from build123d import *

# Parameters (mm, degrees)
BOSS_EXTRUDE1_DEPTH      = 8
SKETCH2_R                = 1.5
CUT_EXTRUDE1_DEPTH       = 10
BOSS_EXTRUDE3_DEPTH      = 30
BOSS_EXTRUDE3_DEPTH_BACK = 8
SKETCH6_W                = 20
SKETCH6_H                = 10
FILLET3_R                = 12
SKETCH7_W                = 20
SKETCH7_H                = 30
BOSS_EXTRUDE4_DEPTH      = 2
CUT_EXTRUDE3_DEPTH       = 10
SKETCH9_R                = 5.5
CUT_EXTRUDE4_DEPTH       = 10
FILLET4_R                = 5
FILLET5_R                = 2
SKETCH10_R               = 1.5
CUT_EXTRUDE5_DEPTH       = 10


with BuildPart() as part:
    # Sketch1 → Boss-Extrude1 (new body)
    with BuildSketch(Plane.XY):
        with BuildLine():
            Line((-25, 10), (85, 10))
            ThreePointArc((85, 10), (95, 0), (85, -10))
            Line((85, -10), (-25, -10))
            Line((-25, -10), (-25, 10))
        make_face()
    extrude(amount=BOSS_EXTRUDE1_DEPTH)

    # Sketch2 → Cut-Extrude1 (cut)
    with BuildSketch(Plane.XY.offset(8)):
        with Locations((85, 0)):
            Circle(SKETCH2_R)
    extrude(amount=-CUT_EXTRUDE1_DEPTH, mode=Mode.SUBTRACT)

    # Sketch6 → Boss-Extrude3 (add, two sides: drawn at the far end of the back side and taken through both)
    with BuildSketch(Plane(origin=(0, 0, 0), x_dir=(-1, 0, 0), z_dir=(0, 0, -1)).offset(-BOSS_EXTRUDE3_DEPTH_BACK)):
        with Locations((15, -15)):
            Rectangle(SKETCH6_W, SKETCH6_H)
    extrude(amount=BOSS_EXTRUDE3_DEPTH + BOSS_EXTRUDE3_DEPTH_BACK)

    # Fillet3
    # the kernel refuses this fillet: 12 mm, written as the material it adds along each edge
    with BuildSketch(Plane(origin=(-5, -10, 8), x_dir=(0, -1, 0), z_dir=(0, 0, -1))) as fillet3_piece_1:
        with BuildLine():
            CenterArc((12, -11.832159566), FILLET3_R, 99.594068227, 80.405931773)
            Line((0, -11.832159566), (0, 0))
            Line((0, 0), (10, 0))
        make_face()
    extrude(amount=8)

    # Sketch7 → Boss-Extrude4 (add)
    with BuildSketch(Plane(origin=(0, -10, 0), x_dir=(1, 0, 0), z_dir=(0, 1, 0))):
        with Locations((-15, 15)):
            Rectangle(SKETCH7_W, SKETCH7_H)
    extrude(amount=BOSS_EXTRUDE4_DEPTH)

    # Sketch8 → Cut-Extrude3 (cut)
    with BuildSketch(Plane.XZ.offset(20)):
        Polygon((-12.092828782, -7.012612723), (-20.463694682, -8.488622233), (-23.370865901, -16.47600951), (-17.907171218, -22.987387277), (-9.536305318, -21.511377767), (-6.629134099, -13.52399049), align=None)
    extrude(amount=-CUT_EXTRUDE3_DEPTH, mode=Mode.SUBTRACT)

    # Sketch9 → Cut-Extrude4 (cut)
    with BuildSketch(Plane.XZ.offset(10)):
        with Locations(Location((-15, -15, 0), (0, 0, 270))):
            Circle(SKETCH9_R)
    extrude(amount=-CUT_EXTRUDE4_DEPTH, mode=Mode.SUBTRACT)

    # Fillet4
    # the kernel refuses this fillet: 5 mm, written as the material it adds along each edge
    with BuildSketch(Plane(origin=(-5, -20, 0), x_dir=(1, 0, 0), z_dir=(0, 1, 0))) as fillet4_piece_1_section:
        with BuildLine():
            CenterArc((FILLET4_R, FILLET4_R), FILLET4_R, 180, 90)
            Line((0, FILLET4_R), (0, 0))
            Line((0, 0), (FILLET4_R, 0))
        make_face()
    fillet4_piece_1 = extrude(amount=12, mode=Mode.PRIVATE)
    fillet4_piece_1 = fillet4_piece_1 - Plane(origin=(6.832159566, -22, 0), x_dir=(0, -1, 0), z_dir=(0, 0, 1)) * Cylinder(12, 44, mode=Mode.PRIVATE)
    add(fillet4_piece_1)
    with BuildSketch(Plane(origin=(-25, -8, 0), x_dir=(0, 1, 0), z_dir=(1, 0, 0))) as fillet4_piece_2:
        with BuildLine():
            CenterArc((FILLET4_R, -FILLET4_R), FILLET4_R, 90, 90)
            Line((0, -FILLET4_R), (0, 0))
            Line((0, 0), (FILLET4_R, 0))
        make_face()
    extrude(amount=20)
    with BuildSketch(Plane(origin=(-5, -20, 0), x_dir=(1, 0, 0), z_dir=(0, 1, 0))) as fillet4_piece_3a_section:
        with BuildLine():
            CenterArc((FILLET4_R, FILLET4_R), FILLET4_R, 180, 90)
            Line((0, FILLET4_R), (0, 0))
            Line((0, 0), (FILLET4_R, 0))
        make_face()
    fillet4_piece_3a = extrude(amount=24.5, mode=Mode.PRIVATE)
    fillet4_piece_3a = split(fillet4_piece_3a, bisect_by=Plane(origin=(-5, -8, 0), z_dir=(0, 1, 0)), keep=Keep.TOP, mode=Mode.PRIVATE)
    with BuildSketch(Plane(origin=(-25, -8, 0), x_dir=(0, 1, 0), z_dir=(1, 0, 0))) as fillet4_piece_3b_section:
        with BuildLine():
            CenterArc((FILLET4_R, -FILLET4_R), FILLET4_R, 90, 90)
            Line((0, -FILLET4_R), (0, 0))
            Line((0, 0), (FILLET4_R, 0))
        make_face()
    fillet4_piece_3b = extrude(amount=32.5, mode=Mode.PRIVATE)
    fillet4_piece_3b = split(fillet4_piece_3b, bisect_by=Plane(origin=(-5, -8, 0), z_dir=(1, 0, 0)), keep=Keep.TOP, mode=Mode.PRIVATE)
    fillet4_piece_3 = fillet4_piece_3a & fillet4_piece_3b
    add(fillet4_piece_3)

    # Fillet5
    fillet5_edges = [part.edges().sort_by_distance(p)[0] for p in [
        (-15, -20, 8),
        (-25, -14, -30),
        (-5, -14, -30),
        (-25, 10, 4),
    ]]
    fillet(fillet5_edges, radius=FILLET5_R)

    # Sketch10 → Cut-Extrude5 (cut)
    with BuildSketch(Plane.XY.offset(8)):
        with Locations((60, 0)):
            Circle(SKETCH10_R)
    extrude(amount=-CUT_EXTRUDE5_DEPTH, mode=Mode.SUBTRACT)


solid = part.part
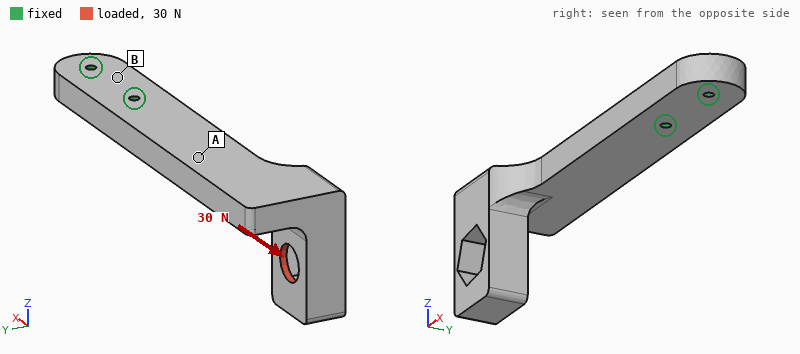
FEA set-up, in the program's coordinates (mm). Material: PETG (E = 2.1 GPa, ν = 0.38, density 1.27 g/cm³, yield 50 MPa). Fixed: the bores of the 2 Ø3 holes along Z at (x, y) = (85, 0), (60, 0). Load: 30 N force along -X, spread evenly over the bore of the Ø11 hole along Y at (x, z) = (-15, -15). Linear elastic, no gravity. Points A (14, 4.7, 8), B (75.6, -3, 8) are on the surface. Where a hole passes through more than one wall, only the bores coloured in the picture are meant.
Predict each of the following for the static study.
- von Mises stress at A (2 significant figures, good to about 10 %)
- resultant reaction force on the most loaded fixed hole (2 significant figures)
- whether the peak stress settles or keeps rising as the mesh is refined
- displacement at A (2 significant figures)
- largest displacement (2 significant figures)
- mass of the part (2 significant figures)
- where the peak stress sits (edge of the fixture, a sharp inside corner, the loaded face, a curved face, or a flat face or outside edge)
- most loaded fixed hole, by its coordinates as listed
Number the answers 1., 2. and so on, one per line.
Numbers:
1. 2.7 MPa
2. 28 N
3. keeps rising
4. 0.37 mm
5. 1.4 mm
6. 33 g
7. edge of the fixture
8. (60, 0)
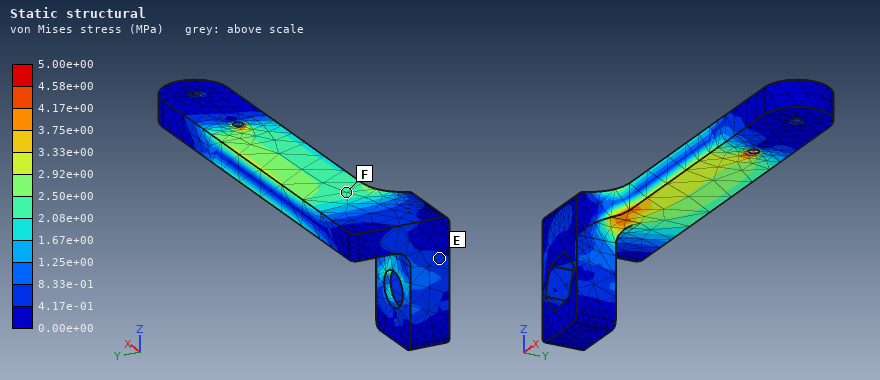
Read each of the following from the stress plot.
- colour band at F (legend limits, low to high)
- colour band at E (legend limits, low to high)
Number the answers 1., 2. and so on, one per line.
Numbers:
1. 2.08e+00 to 2.50e+00 MPa
2. 4.17e-01 to 8.33e-01 MPa
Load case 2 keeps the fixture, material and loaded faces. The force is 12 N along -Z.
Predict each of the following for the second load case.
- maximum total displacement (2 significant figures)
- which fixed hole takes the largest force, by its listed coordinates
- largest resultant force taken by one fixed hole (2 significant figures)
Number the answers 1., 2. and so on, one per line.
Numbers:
1. 1.4 mm
2. (60, 0)
3. 25 N
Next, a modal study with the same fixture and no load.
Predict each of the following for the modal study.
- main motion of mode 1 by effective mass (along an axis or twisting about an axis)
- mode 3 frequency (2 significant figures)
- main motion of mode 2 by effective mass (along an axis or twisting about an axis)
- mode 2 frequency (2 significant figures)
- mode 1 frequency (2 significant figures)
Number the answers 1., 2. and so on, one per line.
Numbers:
1. along Z
2. 510 Hz
3. along Y
4. 270 Hz
5. 130 Hz
